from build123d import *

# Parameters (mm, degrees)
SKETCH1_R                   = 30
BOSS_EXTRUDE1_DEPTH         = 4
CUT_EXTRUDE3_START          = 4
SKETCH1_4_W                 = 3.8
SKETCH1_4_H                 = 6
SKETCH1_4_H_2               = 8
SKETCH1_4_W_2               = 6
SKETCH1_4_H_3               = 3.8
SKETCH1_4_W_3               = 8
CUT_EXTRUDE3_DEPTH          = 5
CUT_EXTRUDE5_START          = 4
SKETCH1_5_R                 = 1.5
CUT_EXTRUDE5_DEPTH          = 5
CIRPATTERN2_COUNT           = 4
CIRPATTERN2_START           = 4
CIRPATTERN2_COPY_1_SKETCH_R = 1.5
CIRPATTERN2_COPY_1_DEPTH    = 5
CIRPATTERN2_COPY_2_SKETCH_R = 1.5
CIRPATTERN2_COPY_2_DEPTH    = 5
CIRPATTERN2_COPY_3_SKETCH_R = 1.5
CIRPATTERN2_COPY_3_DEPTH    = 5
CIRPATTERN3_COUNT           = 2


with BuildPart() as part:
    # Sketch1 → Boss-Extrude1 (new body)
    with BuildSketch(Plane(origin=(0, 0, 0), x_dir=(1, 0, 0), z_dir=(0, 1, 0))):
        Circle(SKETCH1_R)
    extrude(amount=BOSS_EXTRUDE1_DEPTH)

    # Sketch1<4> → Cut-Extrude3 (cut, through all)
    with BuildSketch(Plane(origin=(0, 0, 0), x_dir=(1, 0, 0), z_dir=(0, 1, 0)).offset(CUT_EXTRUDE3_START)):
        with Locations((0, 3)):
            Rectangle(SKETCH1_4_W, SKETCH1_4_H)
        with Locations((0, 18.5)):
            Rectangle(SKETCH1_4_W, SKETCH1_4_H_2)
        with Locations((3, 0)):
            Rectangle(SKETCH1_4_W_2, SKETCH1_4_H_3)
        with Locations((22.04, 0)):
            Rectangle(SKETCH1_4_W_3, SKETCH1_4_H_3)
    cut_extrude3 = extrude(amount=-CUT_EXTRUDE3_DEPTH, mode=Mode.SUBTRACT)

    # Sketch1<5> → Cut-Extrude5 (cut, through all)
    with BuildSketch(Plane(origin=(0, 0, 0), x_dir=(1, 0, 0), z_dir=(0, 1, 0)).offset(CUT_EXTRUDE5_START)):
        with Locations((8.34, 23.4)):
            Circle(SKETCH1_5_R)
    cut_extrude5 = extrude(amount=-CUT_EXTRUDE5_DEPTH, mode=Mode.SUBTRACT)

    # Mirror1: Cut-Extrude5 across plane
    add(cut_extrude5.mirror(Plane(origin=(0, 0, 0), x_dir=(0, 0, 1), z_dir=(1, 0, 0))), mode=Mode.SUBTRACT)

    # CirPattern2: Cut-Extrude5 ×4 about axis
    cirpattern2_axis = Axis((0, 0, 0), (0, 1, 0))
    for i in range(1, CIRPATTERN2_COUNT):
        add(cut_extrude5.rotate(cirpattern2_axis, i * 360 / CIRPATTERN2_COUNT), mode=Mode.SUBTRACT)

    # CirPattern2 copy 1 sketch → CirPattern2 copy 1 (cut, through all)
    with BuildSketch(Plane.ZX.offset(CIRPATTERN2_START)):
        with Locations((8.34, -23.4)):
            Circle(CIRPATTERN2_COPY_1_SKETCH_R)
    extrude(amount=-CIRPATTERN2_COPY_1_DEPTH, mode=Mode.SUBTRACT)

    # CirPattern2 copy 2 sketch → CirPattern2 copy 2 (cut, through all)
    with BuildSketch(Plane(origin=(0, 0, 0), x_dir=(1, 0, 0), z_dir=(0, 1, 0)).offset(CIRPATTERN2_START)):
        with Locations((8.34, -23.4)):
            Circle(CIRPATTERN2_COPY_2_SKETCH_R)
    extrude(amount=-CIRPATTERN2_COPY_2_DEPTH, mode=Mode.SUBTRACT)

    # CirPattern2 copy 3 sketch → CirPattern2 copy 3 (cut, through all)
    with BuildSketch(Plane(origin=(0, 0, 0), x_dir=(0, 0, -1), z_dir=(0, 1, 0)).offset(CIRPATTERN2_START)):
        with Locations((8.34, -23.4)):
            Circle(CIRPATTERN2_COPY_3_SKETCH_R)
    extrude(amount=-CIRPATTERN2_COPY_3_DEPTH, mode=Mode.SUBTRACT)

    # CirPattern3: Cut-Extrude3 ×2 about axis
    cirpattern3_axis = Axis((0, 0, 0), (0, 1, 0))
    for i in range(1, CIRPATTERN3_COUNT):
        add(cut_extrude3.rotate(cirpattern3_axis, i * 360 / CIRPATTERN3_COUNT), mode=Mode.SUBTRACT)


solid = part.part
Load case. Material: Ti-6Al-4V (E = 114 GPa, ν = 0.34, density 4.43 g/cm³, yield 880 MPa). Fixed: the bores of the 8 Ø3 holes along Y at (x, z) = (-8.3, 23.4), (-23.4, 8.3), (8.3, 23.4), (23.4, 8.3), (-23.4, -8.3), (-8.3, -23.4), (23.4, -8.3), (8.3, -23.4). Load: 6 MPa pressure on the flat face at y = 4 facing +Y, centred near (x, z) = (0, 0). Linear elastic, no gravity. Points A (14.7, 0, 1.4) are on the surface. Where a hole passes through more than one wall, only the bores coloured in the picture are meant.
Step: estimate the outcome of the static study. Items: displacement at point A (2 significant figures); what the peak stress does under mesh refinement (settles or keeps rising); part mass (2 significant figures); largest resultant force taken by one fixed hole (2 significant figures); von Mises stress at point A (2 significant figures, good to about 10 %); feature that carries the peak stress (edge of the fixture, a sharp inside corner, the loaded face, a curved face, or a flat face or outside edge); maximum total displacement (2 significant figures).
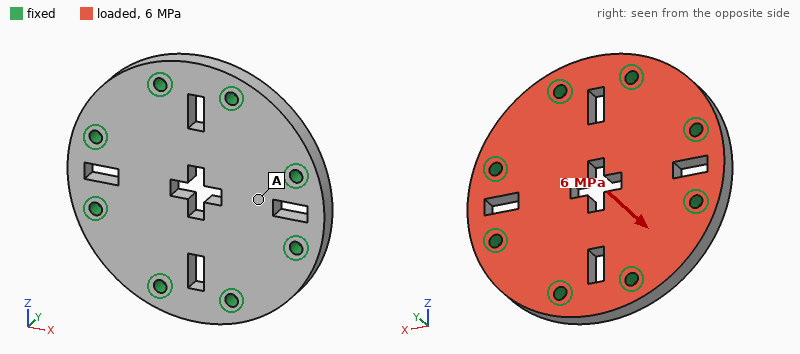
34 µm
keeps rising
46 g
1.9 kN
57 MPa
edge of the fixture
86 µm
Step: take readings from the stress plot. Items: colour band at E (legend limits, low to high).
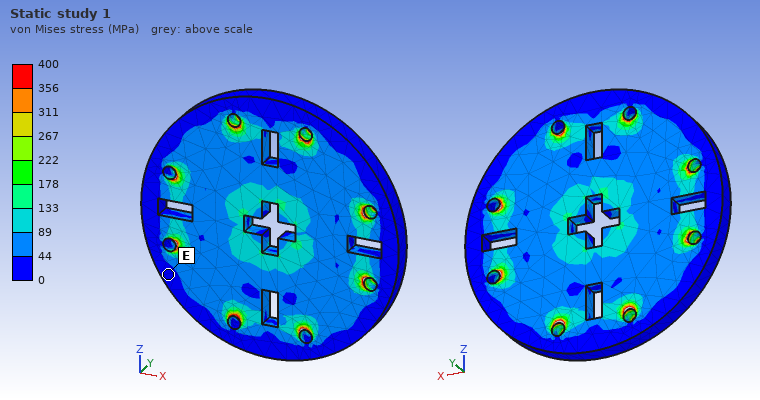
0 to 44 MPa
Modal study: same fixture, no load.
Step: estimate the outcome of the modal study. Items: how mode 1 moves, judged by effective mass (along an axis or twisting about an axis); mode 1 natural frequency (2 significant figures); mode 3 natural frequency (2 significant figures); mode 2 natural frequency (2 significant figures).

along Y
13 kHz
25 kHz
25 kHz
